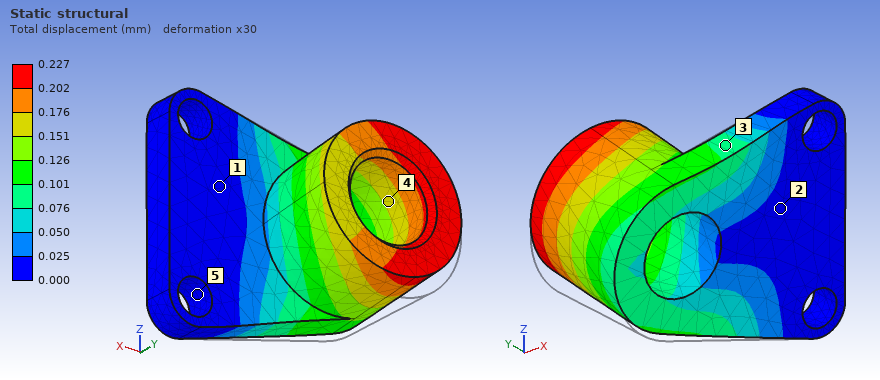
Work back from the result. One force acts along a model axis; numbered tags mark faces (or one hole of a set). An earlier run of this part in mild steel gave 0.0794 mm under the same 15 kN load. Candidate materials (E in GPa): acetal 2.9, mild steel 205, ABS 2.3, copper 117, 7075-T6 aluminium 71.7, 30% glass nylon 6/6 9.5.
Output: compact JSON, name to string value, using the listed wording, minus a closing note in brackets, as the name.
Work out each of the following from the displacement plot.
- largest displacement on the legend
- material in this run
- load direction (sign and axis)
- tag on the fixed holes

{"largest displacement on the legend": "0.227 mm", "material in this run": "7075-T6 aluminium", "load direction": "+Z", "tag on the fixed holes": "5"}
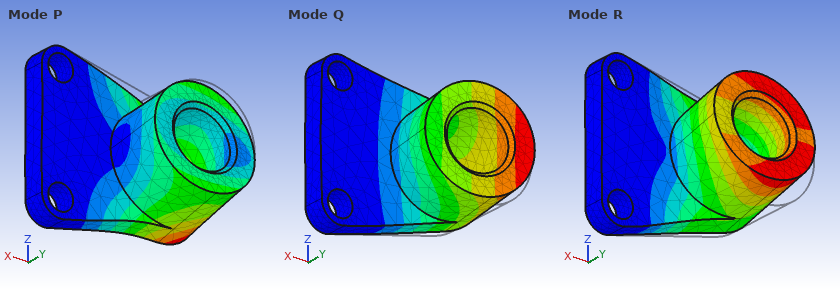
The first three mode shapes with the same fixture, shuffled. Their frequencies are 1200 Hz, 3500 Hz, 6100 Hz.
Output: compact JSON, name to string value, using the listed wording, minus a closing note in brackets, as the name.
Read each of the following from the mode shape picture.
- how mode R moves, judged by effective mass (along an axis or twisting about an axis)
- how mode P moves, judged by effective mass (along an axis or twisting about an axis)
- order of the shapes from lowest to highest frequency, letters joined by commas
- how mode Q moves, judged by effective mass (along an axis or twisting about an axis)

{"how mode R moves, judged by effective mass": "along Z", "how mode P moves, judged by effective mass": "along Z", "order of the shapes from lowest to highest frequency, letters joined by commas": "Q, R, P", "how mode Q moves, judged by effective mass": "along Y"}
